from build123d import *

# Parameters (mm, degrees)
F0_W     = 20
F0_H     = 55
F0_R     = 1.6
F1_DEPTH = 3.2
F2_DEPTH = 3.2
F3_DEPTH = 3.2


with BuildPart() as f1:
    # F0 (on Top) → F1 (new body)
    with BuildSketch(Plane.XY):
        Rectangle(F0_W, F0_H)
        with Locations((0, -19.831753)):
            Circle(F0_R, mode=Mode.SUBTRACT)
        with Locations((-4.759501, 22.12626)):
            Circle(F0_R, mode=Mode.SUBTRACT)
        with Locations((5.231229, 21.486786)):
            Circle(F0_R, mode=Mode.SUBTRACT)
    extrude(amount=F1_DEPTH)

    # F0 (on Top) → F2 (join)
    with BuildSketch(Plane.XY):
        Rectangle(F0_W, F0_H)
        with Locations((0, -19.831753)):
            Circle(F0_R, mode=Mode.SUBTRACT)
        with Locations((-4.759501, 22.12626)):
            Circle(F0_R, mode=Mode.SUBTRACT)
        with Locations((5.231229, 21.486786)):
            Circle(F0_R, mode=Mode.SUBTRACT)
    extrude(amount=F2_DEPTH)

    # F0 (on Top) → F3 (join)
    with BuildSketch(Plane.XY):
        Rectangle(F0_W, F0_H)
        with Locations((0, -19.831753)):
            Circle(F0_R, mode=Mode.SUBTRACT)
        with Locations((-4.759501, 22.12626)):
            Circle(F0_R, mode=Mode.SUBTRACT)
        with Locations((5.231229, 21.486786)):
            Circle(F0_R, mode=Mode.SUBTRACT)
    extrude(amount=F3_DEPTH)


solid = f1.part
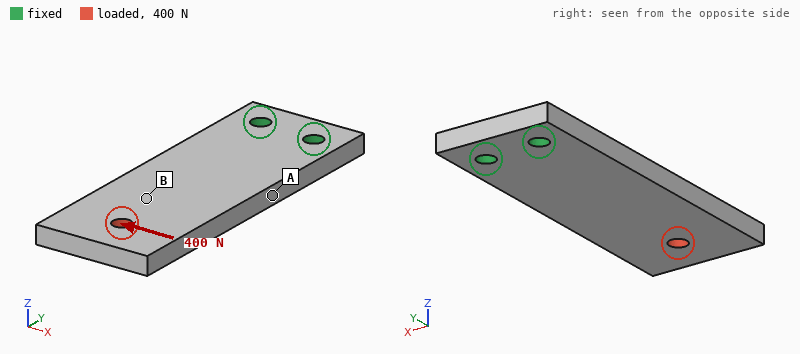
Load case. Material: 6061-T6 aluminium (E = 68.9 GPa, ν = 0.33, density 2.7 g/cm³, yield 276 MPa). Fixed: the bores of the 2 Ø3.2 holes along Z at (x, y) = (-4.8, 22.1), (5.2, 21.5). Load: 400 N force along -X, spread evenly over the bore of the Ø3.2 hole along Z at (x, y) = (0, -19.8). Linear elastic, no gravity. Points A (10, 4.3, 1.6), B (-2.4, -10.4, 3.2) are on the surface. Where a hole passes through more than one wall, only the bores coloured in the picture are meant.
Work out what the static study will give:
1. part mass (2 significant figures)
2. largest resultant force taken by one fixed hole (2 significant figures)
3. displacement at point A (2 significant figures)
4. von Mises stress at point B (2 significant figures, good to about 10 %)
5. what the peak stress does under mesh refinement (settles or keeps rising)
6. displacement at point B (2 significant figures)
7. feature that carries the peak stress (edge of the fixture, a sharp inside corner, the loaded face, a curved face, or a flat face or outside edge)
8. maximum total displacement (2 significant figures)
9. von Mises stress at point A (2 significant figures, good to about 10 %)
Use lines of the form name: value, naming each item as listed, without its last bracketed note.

part mass: 9.3 g
largest resultant force taken by one fixed hole: 1.4 kN
displacement at point A: 0.030 mm
von Mises stress at point B: 16 MPa
what the peak stress does under mesh refinement: keeps rising
displacement at point B: 0.059 mm
feature that carries the peak stress: edge of the fixture
maximum total displacement: 0.11 mm
von Mises stress at point A: 45 MPa
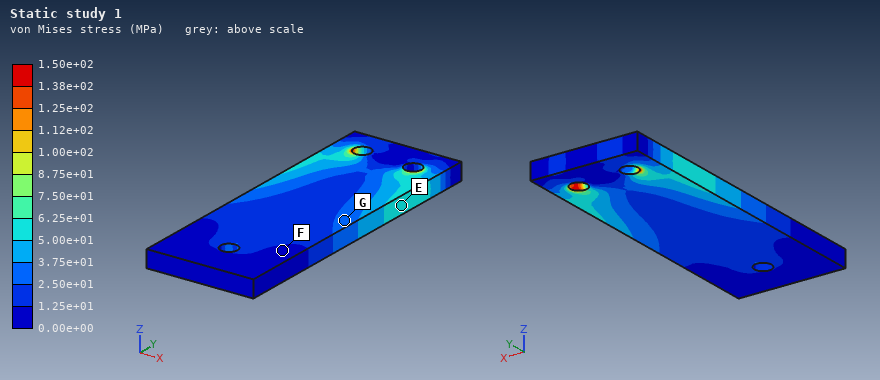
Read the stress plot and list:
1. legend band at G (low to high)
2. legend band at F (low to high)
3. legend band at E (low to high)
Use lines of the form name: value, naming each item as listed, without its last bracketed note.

legend band at G: 2.50e+01 to 3.75e+01 MPa
legend band at F: 0.00e+00 to 1.25e+01 MPa
legend band at E: 5.00e+01 to 6.25e+01 MPa
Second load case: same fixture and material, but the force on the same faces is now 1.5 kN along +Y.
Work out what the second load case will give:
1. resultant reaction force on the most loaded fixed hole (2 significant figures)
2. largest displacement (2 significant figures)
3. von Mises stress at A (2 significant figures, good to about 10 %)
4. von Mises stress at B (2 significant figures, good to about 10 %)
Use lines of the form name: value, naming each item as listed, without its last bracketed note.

resultant reaction force on the most loaded fixed hole: 780 N
largest displacement: 18 µm
von Mises stress at A: 23 MPa
von Mises stress at B: 29 MPa
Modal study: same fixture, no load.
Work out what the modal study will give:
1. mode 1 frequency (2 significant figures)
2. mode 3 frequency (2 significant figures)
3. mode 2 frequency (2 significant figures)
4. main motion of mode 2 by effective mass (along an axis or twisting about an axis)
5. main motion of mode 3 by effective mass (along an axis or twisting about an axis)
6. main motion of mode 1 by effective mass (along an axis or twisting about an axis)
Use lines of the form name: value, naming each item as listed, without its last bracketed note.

mode 1 frequency: 1100 Hz
mode 3 frequency: 5700 Hz
mode 2 frequency: 5200 Hz
main motion of mode 2 by effective mass: twisting about Y
main motion of mode 3 by effective mass: along X
main motion of mode 1 by effective mass: along Z
